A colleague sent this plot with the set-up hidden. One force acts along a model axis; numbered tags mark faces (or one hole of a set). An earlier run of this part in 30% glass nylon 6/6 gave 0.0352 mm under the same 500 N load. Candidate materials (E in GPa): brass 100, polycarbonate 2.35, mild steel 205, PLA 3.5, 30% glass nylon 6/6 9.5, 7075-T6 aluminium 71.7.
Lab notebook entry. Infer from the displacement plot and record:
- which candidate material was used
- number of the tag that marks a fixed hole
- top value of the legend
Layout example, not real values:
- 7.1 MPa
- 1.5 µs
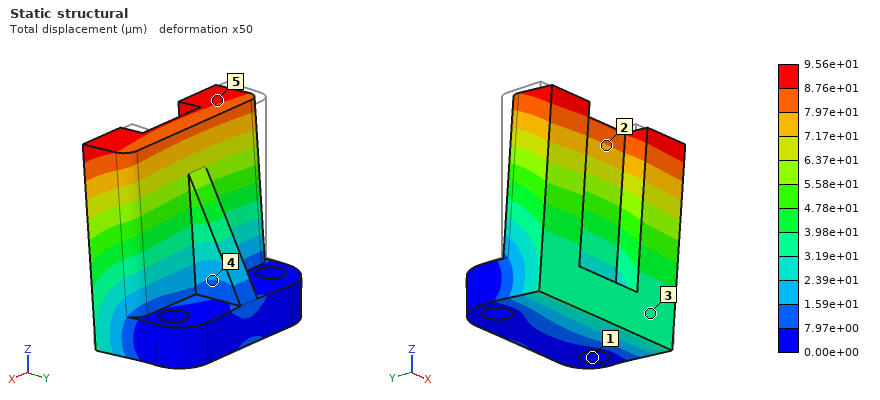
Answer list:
- PLA
- 1
- 9.56e+01 µm
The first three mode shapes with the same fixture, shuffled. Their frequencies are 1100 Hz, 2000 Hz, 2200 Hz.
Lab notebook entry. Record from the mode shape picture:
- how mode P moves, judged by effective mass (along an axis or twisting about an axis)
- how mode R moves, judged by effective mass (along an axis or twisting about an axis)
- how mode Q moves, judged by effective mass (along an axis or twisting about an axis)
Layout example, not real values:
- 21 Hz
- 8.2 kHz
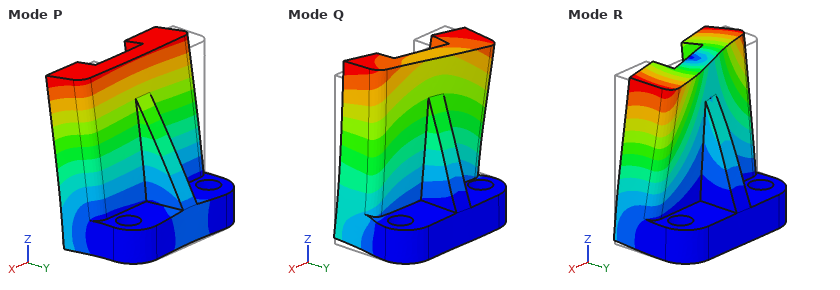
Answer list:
- along Y
- twisting about Z
- along X
